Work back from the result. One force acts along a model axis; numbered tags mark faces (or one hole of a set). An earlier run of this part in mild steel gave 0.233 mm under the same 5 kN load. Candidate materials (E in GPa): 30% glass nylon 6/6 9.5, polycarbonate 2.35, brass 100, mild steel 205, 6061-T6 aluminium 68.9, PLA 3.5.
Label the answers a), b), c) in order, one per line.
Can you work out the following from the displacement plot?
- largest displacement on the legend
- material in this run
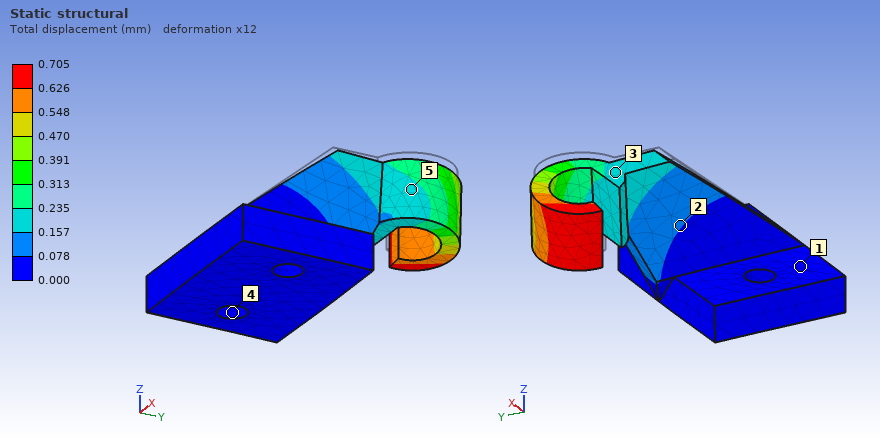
a) 0.705 mm
b) 6061-T6 aluminium
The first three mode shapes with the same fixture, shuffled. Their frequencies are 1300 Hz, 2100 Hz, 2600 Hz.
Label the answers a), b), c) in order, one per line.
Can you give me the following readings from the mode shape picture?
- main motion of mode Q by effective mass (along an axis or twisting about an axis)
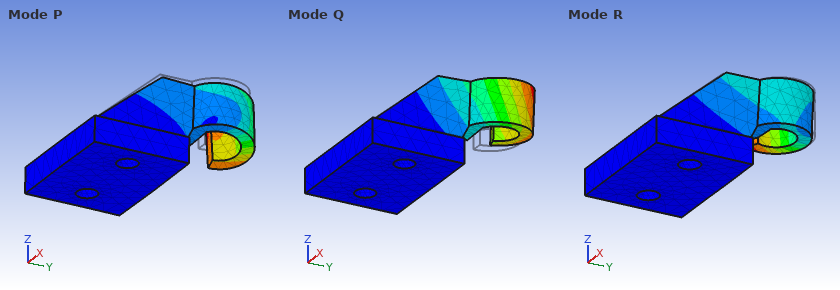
a) along X
